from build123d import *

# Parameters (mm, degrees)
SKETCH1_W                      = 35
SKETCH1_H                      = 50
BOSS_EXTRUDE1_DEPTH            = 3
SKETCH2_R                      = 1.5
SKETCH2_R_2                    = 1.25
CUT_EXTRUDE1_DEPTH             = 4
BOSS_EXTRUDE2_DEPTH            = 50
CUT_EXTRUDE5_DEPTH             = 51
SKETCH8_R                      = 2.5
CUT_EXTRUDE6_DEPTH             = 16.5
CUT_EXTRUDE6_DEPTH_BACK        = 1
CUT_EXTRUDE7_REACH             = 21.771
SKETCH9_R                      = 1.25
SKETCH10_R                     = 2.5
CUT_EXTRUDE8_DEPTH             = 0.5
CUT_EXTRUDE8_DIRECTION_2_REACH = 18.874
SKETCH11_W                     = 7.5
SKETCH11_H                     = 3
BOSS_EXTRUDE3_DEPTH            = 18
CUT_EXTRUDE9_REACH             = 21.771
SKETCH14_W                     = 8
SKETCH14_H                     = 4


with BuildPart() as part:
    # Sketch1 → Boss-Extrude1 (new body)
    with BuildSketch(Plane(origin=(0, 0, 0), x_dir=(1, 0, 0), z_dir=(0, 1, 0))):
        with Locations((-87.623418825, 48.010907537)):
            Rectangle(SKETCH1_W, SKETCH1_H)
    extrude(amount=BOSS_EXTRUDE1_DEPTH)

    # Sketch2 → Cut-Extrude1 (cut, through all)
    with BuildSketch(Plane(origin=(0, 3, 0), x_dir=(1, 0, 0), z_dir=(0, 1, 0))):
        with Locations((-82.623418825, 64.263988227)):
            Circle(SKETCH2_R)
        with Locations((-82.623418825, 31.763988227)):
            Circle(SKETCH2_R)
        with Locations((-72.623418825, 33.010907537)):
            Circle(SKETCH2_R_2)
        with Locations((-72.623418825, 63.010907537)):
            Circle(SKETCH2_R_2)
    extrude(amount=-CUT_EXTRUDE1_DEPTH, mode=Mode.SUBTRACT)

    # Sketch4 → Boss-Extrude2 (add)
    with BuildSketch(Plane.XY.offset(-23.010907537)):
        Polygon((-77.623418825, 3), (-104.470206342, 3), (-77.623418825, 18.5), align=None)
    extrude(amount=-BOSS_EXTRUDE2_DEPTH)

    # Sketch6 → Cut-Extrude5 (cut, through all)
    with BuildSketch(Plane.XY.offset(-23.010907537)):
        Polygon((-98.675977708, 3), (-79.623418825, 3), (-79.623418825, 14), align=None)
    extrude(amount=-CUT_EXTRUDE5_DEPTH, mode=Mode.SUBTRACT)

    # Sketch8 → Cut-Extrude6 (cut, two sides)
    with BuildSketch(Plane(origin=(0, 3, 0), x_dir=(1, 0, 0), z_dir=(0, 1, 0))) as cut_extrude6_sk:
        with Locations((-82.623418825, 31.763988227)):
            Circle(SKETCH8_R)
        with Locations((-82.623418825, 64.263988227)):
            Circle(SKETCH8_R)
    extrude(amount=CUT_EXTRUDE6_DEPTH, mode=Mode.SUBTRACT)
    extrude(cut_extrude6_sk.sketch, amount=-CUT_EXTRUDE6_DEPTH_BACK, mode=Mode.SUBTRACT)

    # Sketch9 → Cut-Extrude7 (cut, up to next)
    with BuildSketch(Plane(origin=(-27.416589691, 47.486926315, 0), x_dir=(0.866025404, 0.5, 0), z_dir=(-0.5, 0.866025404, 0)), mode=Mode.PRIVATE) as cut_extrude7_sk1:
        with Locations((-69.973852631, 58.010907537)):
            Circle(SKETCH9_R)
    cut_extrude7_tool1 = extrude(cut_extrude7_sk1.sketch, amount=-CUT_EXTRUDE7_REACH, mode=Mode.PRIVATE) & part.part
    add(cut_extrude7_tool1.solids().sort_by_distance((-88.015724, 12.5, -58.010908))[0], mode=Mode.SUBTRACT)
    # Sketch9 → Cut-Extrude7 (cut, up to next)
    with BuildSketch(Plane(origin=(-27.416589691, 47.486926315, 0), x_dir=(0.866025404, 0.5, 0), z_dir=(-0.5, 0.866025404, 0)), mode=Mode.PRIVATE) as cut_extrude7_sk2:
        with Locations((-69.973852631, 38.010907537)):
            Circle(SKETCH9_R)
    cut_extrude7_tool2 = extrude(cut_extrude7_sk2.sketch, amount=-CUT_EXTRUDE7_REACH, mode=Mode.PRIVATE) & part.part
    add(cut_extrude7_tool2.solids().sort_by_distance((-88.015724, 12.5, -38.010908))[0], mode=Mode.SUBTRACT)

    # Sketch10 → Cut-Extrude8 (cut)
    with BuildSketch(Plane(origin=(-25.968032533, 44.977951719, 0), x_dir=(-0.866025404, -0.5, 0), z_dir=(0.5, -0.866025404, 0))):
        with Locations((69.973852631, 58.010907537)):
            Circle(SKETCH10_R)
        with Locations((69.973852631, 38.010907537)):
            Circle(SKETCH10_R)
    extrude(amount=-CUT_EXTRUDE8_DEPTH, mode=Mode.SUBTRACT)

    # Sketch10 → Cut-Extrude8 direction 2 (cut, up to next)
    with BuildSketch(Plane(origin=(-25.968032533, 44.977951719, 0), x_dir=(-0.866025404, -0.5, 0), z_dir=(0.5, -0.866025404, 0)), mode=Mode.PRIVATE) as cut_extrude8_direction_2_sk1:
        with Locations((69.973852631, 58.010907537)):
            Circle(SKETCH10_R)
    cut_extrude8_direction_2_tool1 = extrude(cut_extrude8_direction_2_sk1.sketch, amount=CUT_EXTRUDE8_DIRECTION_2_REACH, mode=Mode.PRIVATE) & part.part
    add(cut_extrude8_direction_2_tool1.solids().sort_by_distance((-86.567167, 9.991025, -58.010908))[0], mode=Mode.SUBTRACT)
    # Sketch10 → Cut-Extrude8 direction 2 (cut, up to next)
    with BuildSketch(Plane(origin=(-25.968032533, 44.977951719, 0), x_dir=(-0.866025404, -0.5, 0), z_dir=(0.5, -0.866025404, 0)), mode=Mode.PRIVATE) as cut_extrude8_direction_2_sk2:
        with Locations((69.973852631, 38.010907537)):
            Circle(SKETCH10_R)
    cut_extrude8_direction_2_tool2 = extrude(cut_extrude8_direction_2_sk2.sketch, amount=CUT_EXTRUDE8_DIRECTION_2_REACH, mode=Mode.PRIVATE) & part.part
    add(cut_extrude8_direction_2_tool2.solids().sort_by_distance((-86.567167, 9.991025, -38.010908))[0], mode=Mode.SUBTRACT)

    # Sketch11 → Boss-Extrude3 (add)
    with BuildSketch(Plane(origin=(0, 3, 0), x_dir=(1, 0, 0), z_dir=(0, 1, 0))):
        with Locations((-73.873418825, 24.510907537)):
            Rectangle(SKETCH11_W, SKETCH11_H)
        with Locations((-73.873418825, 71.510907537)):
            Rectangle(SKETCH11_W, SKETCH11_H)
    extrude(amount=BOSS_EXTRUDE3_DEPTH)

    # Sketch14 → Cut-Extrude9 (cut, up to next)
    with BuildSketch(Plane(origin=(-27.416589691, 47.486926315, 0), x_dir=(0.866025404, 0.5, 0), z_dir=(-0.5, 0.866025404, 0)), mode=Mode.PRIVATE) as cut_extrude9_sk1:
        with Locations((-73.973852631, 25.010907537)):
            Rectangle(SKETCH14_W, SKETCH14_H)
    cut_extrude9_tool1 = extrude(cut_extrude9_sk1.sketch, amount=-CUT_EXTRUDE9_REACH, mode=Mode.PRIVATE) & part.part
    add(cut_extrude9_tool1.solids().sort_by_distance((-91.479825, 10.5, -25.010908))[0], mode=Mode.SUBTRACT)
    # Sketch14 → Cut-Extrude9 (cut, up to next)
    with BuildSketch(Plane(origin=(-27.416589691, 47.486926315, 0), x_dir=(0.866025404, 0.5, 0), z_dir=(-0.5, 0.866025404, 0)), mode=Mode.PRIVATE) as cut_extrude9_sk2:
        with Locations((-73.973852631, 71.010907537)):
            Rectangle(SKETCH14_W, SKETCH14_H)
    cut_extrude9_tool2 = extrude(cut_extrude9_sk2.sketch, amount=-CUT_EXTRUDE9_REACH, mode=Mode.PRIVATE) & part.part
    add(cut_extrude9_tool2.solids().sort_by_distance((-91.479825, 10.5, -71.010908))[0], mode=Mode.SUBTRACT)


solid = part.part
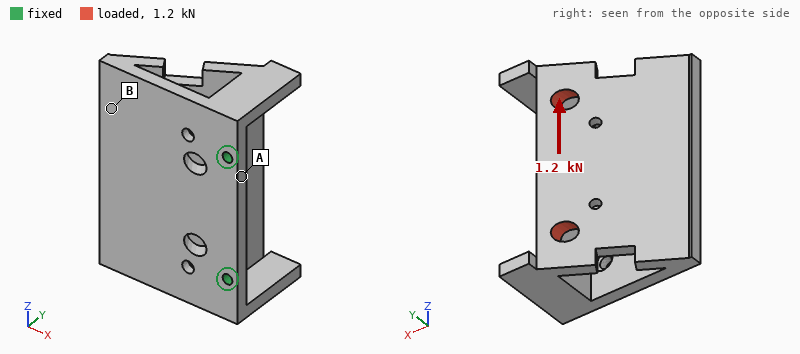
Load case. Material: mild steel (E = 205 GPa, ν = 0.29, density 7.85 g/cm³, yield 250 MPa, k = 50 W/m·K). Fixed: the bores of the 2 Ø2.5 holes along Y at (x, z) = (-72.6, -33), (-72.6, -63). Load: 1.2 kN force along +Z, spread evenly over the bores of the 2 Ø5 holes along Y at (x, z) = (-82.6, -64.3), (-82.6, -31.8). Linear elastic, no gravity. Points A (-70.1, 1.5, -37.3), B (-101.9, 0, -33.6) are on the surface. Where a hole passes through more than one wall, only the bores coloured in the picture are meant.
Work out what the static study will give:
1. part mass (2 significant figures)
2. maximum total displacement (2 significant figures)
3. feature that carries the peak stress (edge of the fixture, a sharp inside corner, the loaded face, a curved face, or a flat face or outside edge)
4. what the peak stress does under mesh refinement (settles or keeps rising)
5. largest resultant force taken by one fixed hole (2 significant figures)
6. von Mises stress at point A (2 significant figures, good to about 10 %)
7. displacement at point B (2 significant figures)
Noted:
83 g
11 µm
edge of the fixture
keeps rising
830 N
16 MPa
6.0 µm
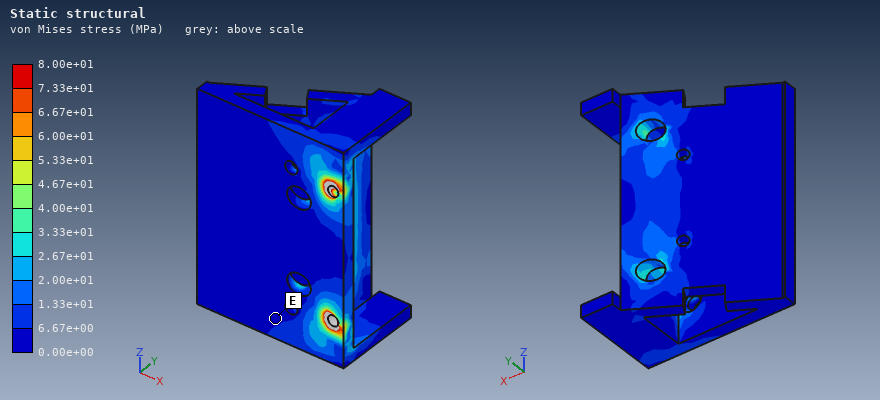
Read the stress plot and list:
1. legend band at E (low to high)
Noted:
0.00e+00 to 6.67e+00 MPa
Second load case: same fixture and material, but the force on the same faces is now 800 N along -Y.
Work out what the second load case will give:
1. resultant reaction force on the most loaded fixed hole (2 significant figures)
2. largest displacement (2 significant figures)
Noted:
400 N
77 µm
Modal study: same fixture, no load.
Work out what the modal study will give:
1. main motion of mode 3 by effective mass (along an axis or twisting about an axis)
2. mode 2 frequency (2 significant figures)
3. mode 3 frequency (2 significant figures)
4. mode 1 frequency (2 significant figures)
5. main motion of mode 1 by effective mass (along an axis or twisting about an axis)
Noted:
along Z
6600 Hz
8800 Hz
1700 Hz
along Y
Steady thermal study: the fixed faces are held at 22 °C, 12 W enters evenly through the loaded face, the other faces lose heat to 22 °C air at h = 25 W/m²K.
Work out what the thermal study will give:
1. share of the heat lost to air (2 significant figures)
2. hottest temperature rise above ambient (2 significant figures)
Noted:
31 %
35 K
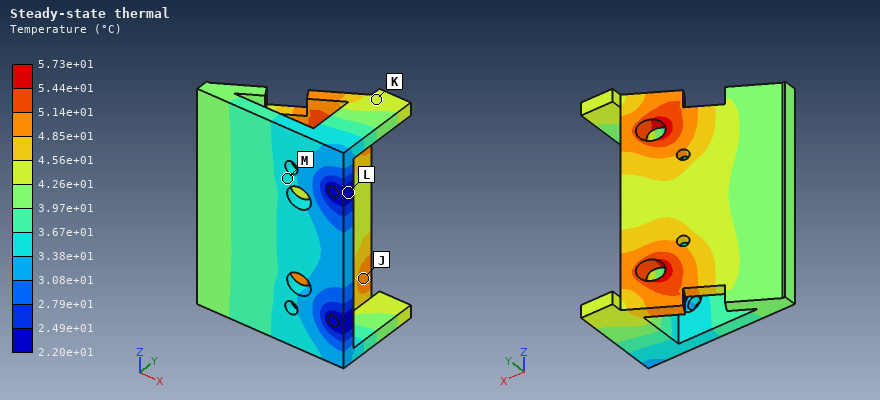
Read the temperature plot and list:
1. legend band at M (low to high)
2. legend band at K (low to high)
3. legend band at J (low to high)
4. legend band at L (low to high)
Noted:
3.38e+01 to 3.67e+01 °C
4.26e+01 to 4.56e+01 °C
4.85e+01 to 5.14e+01 °C
2.20e+01 to 2.49e+01 °C
